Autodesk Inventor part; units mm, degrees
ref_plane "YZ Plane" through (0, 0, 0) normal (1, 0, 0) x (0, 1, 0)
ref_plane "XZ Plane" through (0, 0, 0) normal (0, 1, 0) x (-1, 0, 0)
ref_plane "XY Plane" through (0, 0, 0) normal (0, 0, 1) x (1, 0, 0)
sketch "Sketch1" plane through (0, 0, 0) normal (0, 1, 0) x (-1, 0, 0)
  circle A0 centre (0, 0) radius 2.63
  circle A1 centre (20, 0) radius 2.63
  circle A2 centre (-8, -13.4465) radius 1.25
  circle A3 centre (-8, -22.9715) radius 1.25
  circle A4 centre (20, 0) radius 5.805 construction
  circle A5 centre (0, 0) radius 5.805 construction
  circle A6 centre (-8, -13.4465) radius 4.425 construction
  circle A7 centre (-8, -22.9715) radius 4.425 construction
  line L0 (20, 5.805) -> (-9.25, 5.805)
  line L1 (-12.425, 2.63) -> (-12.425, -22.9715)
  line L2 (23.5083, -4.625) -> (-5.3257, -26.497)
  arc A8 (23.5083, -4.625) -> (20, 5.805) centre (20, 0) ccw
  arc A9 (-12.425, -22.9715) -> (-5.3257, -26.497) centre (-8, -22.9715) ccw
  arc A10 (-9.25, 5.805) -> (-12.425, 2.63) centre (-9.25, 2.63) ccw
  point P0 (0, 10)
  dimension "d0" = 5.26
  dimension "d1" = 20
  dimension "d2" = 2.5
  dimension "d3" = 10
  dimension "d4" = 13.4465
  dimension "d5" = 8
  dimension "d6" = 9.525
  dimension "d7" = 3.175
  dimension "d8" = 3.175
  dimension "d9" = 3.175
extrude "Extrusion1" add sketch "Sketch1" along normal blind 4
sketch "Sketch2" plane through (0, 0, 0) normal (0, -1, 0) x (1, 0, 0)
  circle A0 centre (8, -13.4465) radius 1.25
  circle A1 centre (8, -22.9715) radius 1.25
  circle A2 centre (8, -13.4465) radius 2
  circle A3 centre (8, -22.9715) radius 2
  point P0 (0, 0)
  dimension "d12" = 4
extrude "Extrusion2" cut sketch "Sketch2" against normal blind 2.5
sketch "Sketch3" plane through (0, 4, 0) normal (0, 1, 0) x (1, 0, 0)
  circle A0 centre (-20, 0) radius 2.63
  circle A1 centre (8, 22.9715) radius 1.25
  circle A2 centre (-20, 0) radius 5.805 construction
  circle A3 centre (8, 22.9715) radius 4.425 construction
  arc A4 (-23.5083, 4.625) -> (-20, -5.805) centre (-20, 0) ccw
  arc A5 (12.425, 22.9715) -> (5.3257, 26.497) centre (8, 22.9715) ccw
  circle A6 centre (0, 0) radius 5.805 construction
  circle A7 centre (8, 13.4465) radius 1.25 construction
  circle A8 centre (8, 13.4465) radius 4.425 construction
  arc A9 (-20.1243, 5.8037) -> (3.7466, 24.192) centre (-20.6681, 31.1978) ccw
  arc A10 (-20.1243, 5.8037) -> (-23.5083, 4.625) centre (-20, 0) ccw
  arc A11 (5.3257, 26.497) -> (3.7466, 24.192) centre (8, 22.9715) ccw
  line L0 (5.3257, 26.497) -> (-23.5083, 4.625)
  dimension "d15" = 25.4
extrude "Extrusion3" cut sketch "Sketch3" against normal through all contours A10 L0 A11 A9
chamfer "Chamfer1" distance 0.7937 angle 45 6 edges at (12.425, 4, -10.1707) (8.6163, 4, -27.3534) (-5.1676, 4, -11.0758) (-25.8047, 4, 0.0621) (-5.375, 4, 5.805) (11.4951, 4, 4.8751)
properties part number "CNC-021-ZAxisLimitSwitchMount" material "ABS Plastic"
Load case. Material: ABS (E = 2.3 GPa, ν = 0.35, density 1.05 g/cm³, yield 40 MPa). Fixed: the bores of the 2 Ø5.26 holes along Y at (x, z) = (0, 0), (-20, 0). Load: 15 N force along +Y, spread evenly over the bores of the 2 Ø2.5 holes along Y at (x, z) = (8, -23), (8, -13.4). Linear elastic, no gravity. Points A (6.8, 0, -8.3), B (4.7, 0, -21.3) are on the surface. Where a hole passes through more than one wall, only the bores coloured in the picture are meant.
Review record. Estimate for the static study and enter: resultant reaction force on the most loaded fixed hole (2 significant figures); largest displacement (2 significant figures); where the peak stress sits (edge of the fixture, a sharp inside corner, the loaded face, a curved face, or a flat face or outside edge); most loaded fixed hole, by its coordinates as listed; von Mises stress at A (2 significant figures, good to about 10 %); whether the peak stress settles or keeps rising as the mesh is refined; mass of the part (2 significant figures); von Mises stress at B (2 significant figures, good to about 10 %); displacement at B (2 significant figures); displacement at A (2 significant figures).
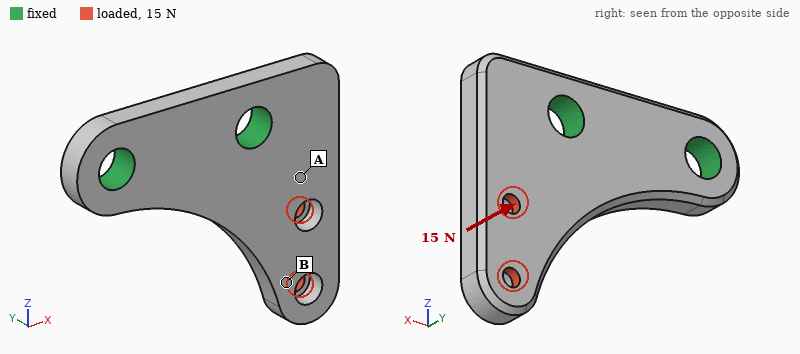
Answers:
18 N
0.28 mm
edge of the fixture
(0, 0)
2.7 MPa
keeps rising
2.7 g
1.1 MPa
0.18 mm
0.048 mm
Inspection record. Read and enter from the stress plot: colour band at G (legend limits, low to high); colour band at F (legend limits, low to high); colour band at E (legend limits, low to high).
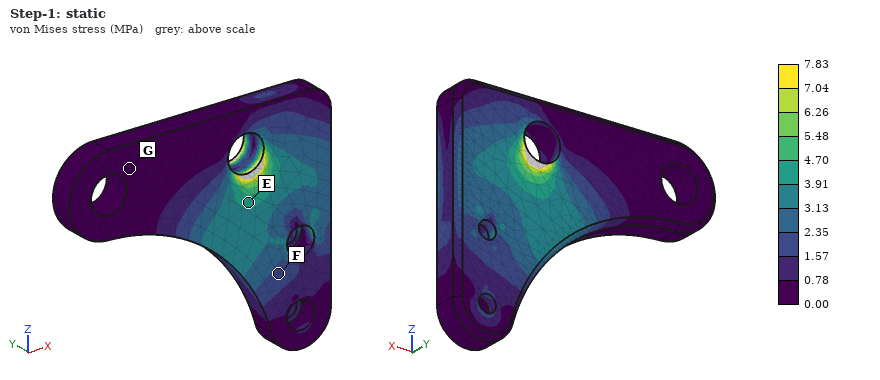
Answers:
0.00 to 0.78 MPa
1.57 to 2.35 MPa
3.91 to 4.70 MPa
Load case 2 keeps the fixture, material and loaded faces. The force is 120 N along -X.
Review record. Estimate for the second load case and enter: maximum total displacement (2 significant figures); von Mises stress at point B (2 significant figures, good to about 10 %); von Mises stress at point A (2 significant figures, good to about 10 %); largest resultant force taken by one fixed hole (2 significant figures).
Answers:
0.26 mm
1.1 MPa
2.4 MPa
95 N
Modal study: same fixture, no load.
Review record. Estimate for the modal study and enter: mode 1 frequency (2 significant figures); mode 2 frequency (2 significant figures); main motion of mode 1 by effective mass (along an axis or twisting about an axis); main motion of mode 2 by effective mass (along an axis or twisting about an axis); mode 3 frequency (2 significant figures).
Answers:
1900 Hz
5200 Hz
along Y
along X
5800 Hz
